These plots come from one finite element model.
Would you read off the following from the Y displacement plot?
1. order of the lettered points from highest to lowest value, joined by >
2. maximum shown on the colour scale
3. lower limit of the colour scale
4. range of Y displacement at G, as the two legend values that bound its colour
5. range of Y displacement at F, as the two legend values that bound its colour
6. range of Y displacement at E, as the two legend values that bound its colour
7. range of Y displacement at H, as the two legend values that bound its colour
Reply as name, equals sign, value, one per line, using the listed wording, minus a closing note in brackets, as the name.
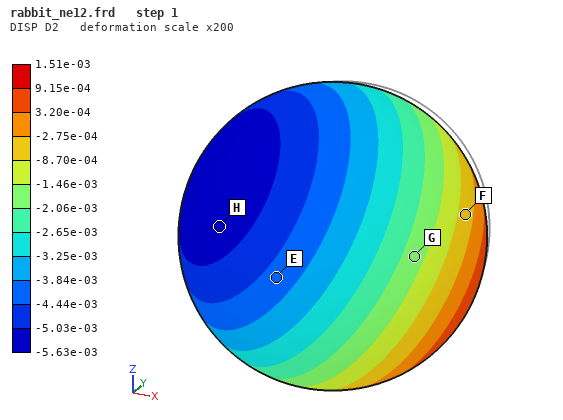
order of the lettered points from highest to lowest value, joined by > = F > G > E > H
maximum shown on the colour scale = 1.51e-03
lower limit of the colour scale = -5.63e-03
range of Y displacement at G, as the two legend values that bound its colour = -2.06e-03 to -1.46e-03
range of Y displacement at F, as the two legend values that bound its colour = -8.70e-04 to -2.75e-04
range of Y displacement at E, as the two legend values that bound its colour = -4.44e-03 to -3.84e-03
range of Y displacement at H, as the two legend values that bound its colour = -5.63e-03 to -5.03e-03
